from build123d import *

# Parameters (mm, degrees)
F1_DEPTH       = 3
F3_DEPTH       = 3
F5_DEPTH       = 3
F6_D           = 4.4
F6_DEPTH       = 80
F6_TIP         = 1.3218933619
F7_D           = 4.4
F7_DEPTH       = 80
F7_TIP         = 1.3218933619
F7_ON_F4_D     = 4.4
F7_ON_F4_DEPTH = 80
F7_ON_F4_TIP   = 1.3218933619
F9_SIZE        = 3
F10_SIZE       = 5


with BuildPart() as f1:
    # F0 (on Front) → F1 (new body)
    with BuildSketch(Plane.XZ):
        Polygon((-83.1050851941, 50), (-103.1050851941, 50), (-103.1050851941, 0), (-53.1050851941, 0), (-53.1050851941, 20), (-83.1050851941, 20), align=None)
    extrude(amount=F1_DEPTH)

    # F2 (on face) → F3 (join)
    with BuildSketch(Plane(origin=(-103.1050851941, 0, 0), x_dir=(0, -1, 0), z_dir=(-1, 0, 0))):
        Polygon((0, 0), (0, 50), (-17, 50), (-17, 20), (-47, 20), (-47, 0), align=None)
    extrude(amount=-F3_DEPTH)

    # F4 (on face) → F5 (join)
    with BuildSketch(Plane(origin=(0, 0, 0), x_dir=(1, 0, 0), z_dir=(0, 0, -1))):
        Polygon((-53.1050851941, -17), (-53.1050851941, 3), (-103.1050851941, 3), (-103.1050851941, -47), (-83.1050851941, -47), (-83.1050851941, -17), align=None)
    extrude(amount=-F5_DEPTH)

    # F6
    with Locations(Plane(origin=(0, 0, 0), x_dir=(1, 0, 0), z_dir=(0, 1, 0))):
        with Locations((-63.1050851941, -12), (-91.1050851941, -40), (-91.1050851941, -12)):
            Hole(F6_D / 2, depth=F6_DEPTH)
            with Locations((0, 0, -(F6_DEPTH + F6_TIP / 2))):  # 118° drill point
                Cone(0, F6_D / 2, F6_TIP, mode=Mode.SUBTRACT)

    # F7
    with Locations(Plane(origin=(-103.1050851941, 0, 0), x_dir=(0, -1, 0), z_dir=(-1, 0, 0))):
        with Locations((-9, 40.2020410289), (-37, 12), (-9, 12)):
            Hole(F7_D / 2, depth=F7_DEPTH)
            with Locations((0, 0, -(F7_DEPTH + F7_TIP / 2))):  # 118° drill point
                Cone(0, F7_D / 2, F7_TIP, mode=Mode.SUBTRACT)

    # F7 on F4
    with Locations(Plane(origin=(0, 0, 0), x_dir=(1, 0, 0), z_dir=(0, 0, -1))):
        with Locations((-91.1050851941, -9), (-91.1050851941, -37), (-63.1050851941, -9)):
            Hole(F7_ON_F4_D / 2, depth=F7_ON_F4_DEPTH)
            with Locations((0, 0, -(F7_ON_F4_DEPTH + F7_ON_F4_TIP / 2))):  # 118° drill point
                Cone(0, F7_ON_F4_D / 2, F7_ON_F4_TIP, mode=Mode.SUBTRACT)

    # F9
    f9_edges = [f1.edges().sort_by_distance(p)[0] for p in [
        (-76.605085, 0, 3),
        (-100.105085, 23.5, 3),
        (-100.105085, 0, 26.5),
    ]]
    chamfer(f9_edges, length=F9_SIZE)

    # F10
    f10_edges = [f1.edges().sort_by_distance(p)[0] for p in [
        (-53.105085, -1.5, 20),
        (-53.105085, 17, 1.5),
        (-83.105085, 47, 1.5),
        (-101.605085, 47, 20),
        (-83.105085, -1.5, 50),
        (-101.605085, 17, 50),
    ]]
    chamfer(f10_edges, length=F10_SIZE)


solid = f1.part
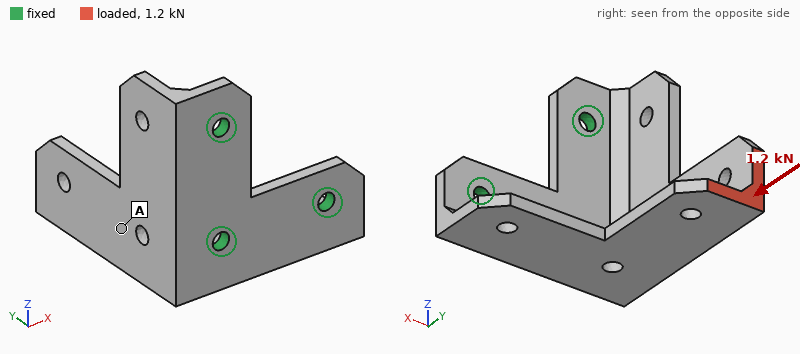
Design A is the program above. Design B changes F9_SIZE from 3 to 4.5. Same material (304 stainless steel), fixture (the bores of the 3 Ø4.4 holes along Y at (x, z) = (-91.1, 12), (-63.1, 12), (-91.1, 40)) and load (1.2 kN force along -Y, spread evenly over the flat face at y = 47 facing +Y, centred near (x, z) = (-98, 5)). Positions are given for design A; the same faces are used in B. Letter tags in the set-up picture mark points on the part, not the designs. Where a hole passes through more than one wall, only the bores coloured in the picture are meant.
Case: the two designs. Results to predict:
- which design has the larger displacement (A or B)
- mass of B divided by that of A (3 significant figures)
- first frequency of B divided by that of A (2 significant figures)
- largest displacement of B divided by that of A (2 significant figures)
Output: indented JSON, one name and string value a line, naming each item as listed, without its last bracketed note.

{
  "which design has the larger displacement": "A",
  "mass of B divided by that of A": "1.06",
  "first frequency of B divided by that of A": "1.1",
  "largest displacement of B divided by that of A": "0.81"
}
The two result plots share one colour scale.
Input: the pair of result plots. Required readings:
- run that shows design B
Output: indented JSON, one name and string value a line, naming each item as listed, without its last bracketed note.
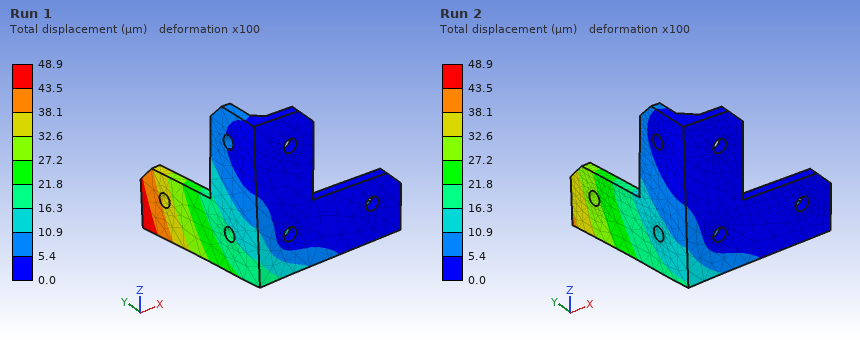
{
  "run that shows design B": "Run 2"
}
